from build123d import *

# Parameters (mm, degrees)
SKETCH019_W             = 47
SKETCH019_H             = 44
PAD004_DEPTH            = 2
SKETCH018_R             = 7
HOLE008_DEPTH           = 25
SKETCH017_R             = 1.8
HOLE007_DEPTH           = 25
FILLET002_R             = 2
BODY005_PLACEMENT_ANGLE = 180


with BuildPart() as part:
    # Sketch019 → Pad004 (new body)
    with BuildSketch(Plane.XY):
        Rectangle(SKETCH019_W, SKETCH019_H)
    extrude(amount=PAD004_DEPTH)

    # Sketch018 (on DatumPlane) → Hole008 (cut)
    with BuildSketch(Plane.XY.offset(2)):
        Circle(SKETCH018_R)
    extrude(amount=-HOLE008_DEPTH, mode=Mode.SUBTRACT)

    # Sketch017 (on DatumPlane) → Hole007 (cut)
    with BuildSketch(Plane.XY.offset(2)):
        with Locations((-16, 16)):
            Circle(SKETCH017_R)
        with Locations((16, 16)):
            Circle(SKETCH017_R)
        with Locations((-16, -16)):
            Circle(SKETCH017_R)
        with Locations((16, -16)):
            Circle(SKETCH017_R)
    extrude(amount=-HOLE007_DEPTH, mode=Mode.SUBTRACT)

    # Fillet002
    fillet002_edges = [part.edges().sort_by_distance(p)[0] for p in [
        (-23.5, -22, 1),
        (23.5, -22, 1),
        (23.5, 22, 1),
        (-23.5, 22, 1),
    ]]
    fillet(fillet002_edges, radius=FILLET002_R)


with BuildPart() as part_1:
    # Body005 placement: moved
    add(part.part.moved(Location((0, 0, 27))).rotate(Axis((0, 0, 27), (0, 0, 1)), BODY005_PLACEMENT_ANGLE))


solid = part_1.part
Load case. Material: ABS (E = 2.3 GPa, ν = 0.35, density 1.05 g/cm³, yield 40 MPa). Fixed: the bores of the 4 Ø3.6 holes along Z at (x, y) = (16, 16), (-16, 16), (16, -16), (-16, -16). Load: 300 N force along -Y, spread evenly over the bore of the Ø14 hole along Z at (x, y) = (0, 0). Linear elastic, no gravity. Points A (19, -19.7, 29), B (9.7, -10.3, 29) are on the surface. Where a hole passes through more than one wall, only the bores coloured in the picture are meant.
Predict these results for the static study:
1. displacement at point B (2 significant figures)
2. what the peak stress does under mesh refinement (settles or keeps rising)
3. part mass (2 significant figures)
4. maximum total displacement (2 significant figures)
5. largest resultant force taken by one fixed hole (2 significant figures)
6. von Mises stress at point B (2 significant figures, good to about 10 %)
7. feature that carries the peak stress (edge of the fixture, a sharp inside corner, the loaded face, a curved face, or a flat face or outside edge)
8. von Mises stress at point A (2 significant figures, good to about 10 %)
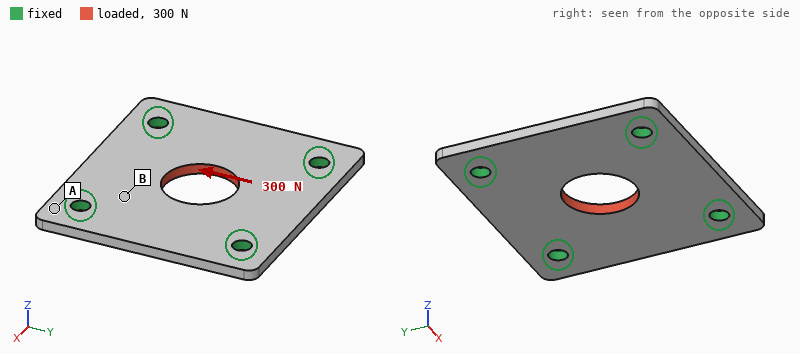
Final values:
18 µm
keeps rising
3.9 g
38 µm
82 N
3.6 MPa
edge of the fixture
1.4 MPa
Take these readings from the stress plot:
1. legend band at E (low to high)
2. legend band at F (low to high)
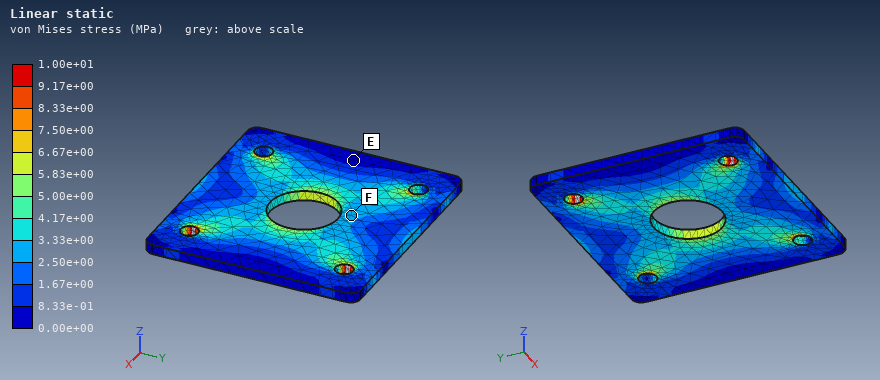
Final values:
0.00e+00 to 8.33e-01 MPa
2.50e+00 to 3.33e+00 MPa
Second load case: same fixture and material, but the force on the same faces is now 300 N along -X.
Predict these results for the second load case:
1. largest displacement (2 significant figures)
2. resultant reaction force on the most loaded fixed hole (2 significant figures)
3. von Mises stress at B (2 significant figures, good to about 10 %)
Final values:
36 µm
80 N
3.5 MPa
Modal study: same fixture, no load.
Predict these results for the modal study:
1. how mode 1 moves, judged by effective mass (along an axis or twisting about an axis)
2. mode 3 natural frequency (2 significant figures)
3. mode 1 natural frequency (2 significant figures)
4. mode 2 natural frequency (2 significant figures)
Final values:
along Z
3300 Hz
2500 Hz
3300 Hz
